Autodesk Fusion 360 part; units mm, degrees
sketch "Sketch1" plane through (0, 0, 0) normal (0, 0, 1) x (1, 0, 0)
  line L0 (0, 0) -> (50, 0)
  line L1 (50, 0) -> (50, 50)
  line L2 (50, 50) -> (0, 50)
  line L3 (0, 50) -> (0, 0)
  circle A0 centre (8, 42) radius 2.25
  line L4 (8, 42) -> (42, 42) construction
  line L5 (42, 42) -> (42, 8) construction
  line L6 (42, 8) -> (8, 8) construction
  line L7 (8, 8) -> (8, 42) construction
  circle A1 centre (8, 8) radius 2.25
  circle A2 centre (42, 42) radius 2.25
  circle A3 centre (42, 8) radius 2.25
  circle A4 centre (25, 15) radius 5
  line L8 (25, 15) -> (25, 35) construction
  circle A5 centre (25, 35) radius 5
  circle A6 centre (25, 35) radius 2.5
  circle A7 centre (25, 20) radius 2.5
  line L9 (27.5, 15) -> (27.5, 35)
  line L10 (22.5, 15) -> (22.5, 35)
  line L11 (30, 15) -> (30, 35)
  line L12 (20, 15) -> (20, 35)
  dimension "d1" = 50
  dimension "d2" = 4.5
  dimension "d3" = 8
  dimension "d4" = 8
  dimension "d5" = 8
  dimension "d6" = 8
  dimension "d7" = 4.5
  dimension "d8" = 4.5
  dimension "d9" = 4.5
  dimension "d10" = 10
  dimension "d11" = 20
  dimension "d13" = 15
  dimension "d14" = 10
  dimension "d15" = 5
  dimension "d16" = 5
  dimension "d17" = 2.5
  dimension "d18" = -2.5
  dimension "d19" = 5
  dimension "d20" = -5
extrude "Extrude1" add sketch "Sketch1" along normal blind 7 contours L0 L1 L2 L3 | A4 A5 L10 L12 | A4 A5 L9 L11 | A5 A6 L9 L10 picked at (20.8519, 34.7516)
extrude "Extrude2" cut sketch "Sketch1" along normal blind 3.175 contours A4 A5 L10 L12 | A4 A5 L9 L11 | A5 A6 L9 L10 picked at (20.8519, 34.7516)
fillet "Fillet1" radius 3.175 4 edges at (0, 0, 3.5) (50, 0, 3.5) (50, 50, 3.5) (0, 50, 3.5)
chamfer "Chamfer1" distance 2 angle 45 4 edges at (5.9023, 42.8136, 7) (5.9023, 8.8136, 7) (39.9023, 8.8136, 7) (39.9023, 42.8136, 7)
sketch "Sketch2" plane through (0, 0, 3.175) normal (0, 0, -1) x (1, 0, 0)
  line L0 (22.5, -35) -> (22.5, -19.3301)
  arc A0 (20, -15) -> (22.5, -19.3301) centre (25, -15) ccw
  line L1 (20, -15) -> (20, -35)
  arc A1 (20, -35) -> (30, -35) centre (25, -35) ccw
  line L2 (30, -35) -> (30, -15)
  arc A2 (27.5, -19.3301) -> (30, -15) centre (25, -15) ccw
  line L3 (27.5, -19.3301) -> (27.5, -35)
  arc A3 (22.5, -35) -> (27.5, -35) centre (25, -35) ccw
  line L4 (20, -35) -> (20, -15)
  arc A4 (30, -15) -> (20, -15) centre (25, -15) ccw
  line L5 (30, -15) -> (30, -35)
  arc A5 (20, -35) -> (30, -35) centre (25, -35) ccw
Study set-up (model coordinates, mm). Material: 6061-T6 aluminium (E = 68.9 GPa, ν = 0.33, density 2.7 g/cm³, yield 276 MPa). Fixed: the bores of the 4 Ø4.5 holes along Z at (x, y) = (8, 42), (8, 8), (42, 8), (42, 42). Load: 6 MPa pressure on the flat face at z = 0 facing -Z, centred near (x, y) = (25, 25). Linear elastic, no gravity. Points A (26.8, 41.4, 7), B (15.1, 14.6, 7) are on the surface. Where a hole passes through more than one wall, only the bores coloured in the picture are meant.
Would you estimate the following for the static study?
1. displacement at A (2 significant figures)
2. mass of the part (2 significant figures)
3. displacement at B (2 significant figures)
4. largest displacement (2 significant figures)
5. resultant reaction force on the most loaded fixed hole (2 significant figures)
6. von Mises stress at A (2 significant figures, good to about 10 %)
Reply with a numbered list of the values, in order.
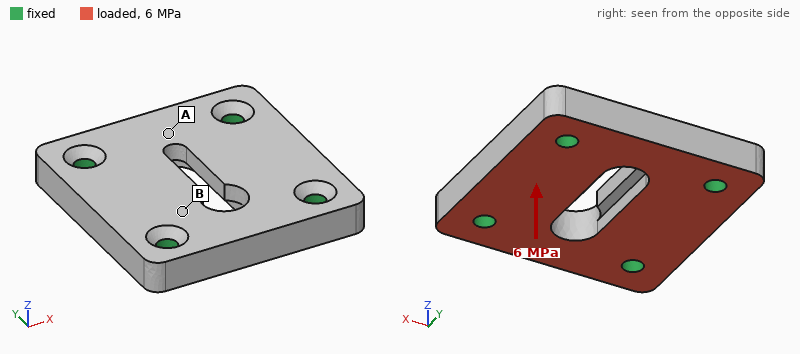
1. 22 µm
2. 41 g
3. 21 µm
4. 39 µm
5. 3.3 kN
6. 46 MPa
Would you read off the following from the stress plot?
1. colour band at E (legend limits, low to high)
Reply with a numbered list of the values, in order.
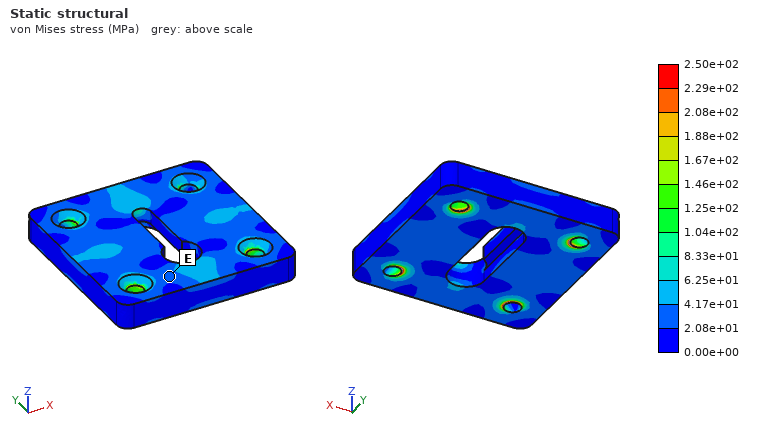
1. 2.08e+01 to 4.17e+01 MPa
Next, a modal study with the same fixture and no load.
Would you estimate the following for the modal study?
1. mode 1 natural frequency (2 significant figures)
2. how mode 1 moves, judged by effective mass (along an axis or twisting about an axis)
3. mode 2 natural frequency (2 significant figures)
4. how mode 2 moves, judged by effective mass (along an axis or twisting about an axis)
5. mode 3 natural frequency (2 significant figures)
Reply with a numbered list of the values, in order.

1. 17 kHz
2. along Z
3. 22 kHz
4. twisting about Y
5. 23 kHz
